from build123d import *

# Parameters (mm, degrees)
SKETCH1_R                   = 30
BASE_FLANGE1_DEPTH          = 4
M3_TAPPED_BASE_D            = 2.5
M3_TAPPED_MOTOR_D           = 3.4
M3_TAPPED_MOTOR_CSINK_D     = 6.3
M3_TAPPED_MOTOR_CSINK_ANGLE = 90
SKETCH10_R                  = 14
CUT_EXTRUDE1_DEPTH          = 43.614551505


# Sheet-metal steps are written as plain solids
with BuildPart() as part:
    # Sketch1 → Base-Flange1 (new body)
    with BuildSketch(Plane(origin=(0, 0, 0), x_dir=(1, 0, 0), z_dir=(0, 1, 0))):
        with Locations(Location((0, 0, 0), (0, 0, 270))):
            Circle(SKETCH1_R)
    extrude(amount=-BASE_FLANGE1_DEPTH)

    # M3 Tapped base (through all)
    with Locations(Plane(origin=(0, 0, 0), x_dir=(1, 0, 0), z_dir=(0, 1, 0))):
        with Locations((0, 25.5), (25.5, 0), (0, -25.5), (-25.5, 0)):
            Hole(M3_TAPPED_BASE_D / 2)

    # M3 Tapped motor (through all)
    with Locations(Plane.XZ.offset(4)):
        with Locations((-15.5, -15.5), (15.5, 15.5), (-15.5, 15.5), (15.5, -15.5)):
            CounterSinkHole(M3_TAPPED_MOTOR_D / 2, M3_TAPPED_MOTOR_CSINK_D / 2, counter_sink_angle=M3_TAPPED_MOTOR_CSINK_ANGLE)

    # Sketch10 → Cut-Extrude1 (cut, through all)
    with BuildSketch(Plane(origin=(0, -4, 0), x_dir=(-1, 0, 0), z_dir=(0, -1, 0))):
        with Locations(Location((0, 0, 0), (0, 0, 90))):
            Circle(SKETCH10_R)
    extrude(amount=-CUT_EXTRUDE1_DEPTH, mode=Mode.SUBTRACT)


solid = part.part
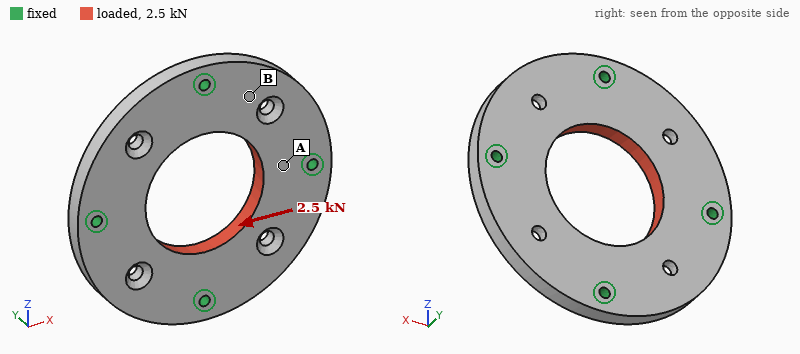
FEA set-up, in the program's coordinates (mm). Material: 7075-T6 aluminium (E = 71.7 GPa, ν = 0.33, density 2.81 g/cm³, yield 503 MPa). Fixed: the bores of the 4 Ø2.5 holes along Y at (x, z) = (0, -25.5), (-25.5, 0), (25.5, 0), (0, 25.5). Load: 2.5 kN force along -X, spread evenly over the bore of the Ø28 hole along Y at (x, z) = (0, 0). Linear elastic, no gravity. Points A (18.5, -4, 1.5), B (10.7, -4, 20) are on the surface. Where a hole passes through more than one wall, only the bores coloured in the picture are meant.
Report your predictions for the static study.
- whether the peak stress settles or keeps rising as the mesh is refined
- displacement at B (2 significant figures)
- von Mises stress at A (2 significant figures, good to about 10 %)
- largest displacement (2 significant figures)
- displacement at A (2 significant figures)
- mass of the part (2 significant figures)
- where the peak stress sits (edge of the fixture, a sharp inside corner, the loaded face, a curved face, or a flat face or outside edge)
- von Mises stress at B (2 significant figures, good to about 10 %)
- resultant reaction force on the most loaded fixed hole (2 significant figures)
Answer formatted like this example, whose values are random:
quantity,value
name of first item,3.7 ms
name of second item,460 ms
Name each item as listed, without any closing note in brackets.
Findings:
quantity,value
whether the peak stress settles or keeps rising as the mesh is refined,keeps rising
displacement at B,2.7 µm
von Mises stress at A,14 MPa
largest displacement,4.2 µm
displacement at A,1.6 µm
mass of the part,24 g
where the peak stress sits,edge of the fixture
von Mises stress at B,5.0 MPa
resultant reaction force on the most loaded fixed hole,660 N
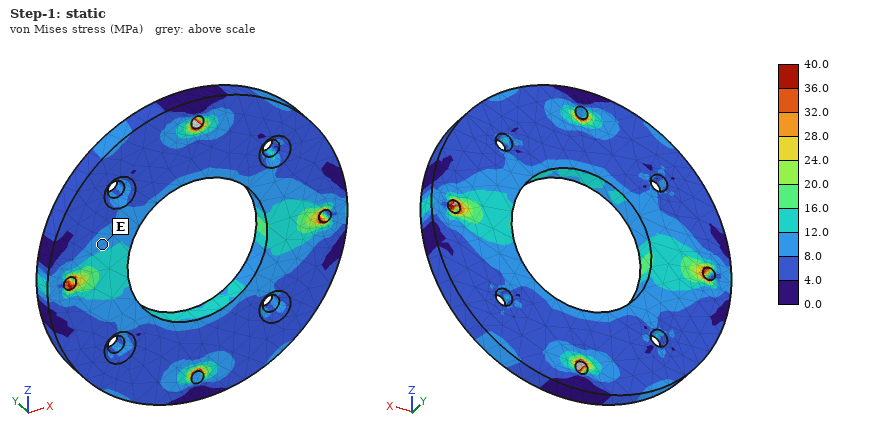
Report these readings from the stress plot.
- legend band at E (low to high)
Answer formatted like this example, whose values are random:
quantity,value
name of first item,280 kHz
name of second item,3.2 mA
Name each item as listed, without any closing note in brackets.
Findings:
quantity,value
legend band at E,8.0 to 12.0 MPa
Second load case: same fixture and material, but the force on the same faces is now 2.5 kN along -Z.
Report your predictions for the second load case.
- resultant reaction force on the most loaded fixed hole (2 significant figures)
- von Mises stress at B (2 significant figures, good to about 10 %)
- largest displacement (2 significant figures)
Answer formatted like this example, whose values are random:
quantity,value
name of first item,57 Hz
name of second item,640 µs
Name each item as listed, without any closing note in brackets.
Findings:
quantity,value
resultant reaction force on the most loaded fixed hole,660 N
von Mises stress at B,6.5 MPa
largest displacement,4.2 µm
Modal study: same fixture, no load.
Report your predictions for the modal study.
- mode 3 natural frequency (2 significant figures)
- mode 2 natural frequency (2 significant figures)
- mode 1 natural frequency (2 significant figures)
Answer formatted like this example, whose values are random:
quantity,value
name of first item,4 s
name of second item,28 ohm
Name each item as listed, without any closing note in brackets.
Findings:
quantity,value
mode 3 natural frequency,12 kHz
mode 2 natural frequency,12 kHz
mode 1 natural frequency,11 kHz
